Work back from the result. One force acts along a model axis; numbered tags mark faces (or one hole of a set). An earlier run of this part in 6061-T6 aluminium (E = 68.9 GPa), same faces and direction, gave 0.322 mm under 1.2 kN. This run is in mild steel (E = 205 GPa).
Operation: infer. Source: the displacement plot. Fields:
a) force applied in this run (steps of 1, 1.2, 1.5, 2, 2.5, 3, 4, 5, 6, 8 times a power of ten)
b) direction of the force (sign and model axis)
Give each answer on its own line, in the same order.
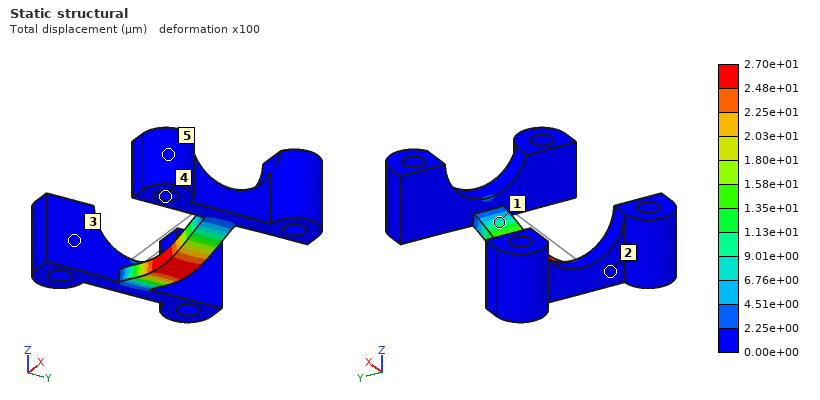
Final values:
300 N
-Z
